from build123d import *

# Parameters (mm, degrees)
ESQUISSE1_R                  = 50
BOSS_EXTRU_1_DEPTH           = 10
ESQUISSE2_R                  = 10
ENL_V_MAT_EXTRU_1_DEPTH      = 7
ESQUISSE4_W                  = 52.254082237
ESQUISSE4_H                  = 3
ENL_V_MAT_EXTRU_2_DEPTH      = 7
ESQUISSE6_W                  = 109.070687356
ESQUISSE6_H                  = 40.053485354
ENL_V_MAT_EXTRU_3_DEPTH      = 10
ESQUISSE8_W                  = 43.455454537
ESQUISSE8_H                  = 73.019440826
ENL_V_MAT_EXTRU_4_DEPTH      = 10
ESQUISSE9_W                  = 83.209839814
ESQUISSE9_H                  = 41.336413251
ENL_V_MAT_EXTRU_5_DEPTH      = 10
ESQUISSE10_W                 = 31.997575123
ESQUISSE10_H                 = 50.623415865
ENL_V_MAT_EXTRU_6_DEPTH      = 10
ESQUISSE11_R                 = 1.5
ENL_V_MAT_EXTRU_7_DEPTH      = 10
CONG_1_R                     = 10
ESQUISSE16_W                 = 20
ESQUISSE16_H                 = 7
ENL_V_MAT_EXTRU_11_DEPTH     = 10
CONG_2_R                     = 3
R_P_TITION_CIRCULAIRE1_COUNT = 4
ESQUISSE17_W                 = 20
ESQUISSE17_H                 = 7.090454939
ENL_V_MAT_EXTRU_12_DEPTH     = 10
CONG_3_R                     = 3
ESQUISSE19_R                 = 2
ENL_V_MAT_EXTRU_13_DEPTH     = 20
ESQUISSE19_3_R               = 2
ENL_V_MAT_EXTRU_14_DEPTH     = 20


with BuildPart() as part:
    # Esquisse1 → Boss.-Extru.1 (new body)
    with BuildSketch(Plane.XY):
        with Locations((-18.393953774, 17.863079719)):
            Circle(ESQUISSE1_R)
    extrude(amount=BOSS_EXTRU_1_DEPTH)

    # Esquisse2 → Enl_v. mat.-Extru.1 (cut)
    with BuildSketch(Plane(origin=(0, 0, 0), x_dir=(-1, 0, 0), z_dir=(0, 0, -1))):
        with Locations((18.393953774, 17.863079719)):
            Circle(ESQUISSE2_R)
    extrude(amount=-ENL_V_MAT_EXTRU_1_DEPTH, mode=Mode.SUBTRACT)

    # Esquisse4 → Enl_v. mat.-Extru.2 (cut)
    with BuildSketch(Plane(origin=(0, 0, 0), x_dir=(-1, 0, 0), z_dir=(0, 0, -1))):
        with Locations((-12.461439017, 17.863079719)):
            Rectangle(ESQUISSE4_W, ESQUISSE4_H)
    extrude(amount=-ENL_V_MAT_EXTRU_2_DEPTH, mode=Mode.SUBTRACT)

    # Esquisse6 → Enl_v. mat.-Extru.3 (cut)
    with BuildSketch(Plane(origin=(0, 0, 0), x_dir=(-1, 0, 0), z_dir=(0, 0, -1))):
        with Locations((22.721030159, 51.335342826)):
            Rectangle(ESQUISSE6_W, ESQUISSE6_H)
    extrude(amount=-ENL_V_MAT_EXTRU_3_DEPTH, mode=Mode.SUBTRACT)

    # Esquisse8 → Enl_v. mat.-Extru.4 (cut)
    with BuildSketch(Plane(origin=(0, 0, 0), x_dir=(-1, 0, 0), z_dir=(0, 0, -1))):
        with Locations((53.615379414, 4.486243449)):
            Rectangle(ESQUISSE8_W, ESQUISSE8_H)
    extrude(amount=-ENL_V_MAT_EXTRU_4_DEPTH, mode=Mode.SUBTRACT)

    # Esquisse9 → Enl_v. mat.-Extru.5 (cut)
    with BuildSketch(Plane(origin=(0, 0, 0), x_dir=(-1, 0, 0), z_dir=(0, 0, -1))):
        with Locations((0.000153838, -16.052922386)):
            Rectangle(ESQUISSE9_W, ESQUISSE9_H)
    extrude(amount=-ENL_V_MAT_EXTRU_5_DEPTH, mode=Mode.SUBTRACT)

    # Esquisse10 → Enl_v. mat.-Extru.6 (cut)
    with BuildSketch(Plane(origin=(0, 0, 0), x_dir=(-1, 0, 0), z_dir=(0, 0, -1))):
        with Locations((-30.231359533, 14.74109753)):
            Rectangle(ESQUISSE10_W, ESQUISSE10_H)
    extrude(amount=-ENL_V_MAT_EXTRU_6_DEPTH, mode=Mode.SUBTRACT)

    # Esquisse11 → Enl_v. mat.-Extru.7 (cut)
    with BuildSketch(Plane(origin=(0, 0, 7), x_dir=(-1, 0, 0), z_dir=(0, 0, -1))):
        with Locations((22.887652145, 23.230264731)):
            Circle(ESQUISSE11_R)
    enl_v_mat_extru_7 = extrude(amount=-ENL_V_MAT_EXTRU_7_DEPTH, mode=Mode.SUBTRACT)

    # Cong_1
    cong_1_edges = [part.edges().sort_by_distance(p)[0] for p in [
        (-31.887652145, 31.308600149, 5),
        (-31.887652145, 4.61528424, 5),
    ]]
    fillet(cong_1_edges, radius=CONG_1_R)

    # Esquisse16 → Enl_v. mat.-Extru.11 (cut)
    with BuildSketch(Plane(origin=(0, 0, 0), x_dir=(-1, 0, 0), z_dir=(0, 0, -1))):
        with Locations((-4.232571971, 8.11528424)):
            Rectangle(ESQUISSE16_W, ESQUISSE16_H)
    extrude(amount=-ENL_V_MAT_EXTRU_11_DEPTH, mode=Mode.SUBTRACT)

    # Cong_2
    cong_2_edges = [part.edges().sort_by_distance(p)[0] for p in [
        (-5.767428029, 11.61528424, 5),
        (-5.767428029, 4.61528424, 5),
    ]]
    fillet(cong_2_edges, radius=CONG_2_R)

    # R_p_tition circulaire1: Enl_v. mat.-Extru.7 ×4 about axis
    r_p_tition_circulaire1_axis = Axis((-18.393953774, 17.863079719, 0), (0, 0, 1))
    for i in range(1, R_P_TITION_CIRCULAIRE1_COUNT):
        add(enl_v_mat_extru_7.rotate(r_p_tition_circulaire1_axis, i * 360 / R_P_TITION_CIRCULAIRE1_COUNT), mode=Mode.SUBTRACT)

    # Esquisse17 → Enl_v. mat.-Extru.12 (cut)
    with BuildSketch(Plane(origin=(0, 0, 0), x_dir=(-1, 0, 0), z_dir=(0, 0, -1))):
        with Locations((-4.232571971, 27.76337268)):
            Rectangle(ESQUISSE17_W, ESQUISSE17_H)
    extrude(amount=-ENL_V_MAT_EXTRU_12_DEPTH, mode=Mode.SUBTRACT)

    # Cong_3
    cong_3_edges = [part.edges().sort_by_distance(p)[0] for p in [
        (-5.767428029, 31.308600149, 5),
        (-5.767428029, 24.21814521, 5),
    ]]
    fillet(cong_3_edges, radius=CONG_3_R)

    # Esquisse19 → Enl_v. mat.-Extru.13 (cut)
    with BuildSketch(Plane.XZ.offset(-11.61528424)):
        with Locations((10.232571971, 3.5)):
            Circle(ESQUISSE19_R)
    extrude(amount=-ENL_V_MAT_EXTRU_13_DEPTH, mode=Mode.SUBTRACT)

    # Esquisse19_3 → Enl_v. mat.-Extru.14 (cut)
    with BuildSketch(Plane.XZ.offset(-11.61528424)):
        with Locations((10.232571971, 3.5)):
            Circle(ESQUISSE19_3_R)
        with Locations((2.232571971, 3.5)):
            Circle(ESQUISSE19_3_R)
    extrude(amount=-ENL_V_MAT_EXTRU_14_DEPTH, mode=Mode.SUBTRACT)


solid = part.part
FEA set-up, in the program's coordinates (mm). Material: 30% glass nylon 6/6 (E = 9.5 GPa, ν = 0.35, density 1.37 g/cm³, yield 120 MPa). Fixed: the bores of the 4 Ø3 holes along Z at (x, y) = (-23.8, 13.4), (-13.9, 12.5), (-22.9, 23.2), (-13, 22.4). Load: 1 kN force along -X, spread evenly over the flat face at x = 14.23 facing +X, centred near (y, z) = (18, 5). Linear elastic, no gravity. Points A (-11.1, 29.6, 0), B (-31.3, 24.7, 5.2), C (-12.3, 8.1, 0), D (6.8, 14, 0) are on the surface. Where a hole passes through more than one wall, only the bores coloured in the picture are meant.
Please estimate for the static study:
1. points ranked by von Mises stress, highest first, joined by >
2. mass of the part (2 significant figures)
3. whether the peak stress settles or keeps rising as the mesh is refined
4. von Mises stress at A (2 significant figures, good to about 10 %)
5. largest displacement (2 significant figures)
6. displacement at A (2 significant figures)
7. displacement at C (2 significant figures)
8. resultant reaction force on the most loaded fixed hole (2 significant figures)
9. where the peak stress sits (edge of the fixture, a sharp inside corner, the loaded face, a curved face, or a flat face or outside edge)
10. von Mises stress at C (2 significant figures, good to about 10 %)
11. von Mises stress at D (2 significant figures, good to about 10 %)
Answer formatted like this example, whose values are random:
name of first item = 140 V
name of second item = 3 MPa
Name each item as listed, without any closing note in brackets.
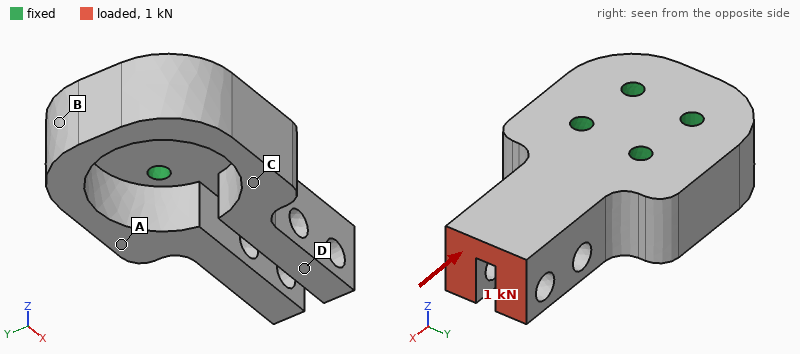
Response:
points ranked by von Mises stress, highest first, joined by > = D > C > A > B
mass of the part = 8.3 g
whether the peak stress settles or keeps rising as the mesh is refined = keeps rising
von Mises stress at A = 9.2 MPa
largest displacement = 0.20 mm
displacement at A = 0.036 mm
displacement at C = 0.038 mm
resultant reaction force on the most loaded fixed hole = 450 N
where the peak stress sits = edge of the fixture
von Mises stress at C = 14 MPa
von Mises stress at D = 23 MPa
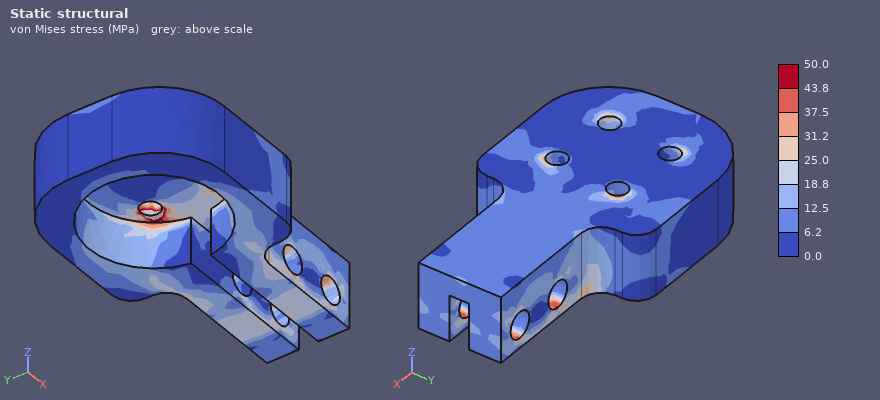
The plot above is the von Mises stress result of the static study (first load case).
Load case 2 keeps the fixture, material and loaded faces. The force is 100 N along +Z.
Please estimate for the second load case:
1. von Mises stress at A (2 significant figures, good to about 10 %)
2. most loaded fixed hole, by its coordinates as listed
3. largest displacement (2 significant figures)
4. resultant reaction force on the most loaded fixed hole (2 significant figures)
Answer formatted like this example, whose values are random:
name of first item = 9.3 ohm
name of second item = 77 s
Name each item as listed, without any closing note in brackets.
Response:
von Mises stress at A = 8.4 MPa
most loaded fixed hole, by its coordinates as listed = (-13, 22.4)
largest displacement = 0.21 mm
resultant reaction force on the most loaded fixed hole = 160 N
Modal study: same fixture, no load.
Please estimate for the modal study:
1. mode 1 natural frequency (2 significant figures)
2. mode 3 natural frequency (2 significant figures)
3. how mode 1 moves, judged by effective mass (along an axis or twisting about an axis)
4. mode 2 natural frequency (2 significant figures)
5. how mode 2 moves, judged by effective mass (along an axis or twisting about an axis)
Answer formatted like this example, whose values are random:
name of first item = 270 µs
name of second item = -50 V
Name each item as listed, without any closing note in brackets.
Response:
mode 1 natural frequency = 3500 Hz
mode 3 natural frequency = 8000 Hz
how mode 1 moves, judged by effective mass = along Z
mode 2 natural frequency = 6100 Hz
how mode 2 moves, judged by effective mass = along Y
